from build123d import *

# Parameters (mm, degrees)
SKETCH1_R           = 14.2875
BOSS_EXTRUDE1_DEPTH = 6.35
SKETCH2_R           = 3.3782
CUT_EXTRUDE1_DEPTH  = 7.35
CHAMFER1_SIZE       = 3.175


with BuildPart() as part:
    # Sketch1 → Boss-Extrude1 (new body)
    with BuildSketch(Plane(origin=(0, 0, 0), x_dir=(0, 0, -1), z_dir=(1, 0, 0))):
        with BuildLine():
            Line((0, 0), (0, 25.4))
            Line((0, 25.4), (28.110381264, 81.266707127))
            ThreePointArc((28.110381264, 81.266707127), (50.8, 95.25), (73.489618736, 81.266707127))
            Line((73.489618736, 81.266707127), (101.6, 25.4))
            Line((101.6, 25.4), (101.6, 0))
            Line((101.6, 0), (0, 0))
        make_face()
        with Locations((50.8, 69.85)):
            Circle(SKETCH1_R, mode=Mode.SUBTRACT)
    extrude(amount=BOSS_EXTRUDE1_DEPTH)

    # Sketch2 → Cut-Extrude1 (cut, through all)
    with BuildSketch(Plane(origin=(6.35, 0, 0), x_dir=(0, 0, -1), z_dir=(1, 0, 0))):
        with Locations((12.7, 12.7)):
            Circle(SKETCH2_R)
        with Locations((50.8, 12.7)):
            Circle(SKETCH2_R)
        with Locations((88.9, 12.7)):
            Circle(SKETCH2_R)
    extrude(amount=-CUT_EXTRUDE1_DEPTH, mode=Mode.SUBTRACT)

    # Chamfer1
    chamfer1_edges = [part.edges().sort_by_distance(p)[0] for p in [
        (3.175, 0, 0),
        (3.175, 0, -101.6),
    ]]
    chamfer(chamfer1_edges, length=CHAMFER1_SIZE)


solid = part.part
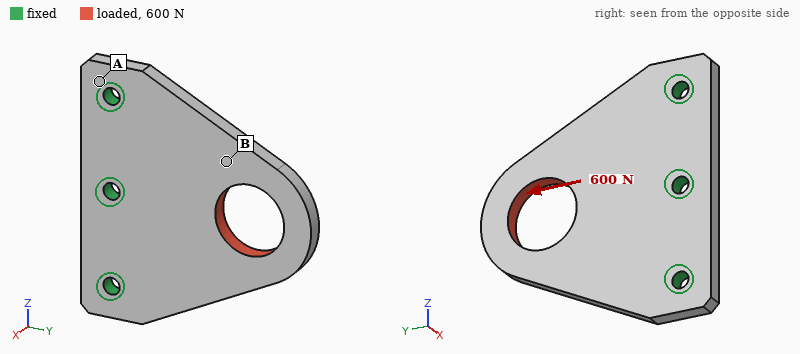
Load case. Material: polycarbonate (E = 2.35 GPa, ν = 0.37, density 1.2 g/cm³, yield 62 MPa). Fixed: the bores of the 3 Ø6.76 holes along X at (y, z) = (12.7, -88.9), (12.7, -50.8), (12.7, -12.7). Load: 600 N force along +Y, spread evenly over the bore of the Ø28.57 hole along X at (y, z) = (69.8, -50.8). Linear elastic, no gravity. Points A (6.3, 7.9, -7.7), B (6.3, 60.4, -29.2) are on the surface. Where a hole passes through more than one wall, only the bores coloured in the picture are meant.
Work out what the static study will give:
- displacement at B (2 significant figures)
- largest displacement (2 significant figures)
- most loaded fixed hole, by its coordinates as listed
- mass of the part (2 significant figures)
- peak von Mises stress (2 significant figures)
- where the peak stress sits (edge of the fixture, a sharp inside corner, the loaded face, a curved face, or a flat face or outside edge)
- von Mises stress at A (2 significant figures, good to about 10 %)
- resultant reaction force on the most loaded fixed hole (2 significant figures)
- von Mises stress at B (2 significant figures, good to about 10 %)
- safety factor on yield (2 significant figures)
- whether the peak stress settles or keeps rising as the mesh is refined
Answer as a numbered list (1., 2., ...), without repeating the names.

1. 29 µm
2. 74 µm
3. (12.7, -50.8)
4. 49 g
5. 4.4 MPa
6. the loaded face
7. 0.60 MPa
8. 230 N
9. 1.9 MPa
10. 14
11. settles
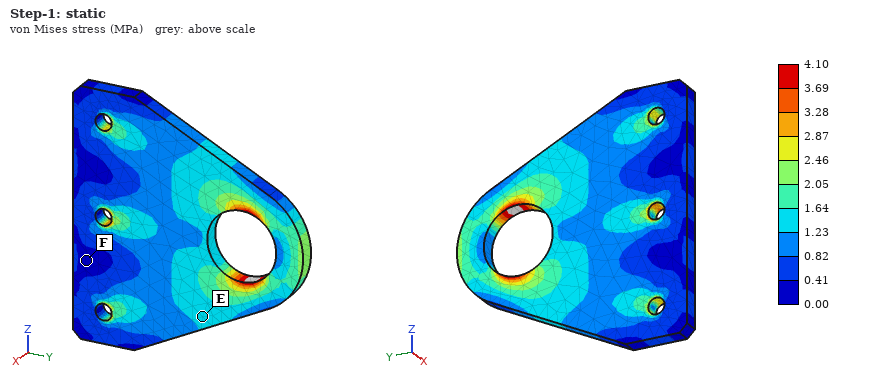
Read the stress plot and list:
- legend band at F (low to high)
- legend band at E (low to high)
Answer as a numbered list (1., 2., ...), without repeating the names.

1. 0.00 to 0.41 MPa
2. 1.23 to 1.64 MPa
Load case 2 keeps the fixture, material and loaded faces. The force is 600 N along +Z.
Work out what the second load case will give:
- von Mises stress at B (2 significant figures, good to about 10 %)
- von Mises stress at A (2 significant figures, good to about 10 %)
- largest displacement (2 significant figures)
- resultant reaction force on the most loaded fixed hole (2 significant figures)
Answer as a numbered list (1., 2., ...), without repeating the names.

1. 2.0 MPa
2. 1.8 MPa
3. 0.24 mm
4. 470 N
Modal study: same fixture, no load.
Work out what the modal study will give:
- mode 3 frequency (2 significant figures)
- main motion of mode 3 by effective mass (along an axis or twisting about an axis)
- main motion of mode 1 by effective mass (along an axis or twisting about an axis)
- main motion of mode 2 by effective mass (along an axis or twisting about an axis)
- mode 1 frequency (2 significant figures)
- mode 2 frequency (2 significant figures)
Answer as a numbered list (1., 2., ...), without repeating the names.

1. 1300 Hz
2. along X
3. along X
4. twisting about Y
5. 340 Hz
6. 890 Hz
